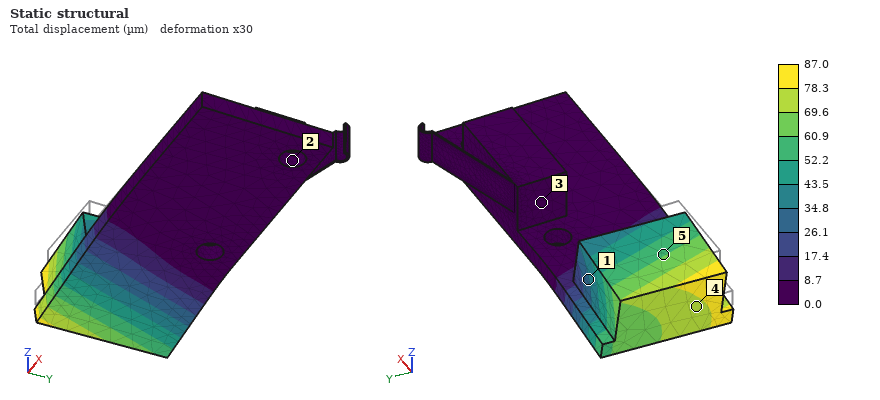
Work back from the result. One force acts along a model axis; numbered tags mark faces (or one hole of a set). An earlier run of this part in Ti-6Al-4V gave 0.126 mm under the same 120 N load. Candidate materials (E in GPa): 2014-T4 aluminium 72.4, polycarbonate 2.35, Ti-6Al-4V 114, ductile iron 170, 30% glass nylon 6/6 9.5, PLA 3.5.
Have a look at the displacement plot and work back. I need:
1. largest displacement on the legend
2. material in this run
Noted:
87.0 µm
ductile iron
